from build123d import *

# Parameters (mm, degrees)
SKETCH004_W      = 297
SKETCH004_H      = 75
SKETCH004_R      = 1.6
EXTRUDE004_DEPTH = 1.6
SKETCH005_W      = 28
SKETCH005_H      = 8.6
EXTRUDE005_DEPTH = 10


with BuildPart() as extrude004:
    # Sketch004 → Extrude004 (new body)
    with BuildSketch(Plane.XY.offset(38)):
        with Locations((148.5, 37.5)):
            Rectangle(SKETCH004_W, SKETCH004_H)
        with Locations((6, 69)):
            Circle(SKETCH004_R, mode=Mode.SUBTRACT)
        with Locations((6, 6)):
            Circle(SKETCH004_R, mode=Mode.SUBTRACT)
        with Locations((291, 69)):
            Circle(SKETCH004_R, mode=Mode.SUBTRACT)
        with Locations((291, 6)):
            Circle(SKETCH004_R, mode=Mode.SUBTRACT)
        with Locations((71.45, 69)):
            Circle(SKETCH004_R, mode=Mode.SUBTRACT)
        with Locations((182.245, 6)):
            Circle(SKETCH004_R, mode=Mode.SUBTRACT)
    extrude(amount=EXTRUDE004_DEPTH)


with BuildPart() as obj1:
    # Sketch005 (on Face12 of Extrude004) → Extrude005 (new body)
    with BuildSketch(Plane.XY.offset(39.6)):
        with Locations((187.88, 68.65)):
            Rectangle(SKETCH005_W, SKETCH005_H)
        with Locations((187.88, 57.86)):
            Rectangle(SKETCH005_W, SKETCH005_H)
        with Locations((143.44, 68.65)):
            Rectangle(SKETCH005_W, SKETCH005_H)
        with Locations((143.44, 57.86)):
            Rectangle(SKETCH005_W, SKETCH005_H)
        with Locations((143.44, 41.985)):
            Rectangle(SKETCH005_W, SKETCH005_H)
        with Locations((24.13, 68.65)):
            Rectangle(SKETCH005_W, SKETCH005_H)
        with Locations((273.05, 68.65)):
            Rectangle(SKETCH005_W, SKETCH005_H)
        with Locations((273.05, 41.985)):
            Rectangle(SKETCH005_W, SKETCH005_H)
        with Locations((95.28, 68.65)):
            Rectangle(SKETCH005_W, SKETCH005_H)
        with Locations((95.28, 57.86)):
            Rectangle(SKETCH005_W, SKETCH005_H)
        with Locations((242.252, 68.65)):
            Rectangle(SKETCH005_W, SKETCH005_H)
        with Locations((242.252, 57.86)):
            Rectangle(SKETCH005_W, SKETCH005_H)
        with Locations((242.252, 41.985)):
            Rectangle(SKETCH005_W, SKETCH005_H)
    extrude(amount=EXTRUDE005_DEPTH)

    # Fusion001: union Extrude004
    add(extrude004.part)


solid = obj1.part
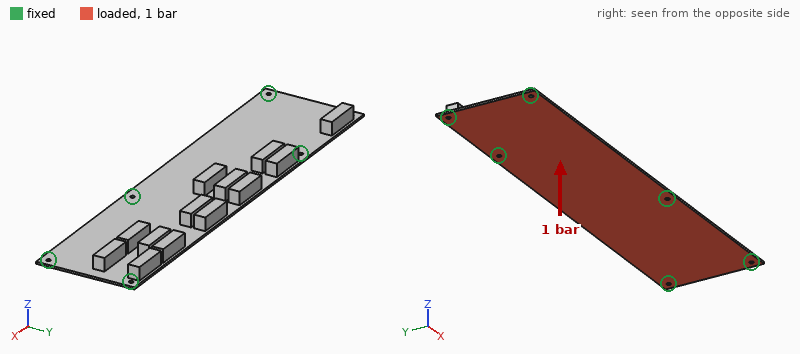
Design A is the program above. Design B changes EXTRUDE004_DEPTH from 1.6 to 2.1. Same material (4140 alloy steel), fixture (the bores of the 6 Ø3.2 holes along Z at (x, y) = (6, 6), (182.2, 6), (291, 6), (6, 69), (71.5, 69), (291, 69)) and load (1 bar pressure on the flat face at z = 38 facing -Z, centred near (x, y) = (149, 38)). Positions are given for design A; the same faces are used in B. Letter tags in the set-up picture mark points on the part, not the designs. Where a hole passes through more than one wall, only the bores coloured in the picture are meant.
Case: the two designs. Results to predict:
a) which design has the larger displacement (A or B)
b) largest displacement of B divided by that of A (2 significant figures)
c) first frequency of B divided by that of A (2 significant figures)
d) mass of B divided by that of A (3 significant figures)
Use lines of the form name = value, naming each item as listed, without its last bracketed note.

which design has the larger displacement = A
largest displacement of B divided by that of A = 0.47
first frequency of B divided by that of A = 1.4
mass of B divided by that of A = 1.14
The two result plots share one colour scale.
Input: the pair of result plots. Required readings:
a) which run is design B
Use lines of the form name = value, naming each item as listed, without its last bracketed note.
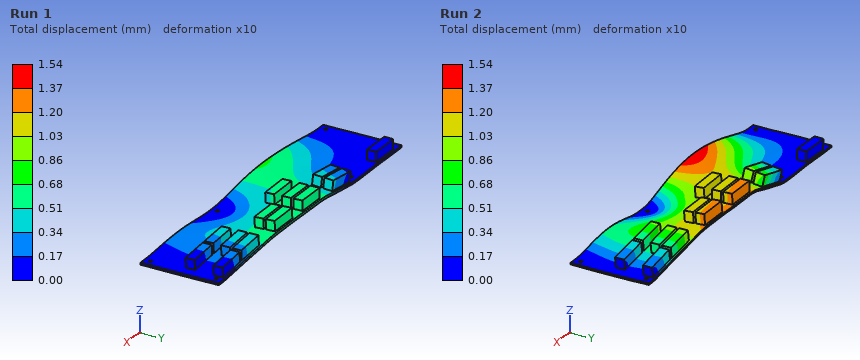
which run is design B = Run 1
